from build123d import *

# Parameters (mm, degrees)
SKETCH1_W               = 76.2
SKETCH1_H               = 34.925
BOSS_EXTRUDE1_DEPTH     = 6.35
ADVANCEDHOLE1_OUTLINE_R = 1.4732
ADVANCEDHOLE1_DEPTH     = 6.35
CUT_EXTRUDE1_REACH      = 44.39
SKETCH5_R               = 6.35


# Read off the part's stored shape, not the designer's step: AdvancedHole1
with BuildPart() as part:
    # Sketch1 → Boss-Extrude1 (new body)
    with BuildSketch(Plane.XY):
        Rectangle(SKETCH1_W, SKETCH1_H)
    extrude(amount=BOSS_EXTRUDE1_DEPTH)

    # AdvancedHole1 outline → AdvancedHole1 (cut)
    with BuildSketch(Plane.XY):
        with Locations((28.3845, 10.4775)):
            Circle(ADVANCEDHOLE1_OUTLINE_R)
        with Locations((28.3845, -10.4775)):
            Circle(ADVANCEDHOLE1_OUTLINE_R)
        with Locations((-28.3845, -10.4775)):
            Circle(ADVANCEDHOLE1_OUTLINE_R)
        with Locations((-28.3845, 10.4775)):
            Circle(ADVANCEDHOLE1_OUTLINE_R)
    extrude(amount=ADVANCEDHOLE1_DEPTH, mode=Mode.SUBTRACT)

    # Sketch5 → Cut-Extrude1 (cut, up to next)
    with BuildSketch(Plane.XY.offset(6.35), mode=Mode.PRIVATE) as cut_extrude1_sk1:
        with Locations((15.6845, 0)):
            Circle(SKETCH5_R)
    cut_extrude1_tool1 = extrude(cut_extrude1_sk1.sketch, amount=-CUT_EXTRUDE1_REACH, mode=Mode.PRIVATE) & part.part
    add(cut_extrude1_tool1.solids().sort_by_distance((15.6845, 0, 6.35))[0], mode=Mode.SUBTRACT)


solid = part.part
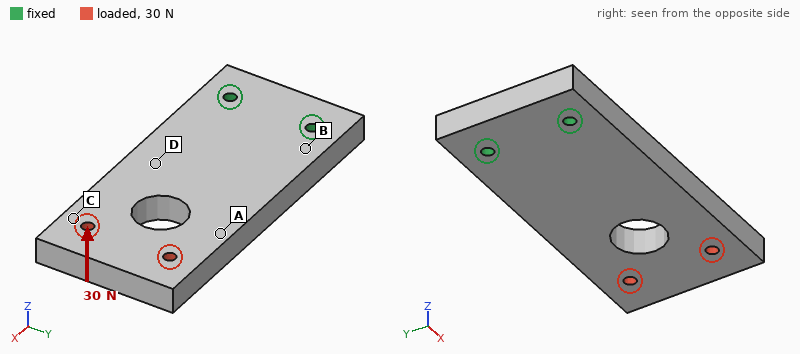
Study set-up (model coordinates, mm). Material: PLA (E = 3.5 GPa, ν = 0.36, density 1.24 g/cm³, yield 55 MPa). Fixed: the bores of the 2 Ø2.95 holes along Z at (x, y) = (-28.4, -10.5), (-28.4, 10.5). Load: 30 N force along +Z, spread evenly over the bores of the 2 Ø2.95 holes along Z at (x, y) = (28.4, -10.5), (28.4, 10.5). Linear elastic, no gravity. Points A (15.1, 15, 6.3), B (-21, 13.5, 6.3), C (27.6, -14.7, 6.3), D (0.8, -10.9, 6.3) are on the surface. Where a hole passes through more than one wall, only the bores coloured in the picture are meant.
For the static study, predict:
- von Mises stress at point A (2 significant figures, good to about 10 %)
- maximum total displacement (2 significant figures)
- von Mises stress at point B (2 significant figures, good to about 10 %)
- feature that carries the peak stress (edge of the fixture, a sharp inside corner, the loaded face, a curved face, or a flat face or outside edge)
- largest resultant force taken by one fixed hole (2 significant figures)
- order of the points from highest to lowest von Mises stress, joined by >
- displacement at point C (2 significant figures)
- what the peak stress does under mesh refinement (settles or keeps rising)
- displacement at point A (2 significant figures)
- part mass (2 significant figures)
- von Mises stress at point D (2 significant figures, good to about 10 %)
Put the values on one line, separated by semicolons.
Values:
2.4 MPa; 0.97 mm; 6.4 MPa; edge of the fixture; 15 N; B > D > A > C; 0.75 mm; keeps rising; 0.50 mm; 20 g; 3.7 MPa
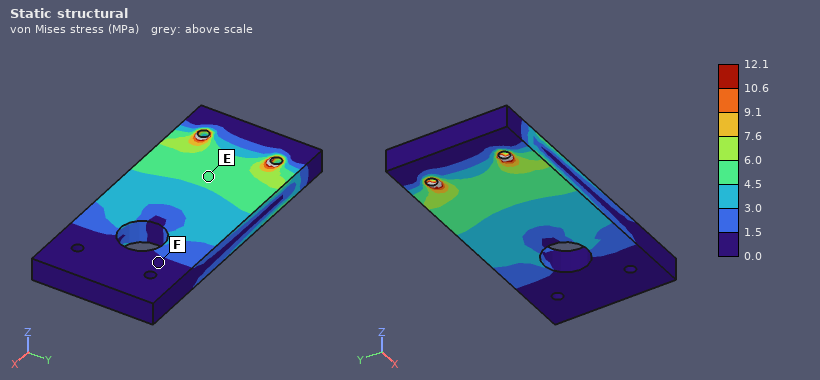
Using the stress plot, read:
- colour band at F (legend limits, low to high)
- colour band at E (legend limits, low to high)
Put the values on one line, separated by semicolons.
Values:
0.0 to 1.5 MPa; 4.5 to 6.0 MPa
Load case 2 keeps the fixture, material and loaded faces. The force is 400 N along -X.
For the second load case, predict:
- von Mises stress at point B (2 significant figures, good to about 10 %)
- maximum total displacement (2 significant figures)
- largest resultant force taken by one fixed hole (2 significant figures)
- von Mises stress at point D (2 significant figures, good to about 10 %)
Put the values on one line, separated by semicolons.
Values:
2.1 MPa; 42 µm; 200 N; 2.1 MPa
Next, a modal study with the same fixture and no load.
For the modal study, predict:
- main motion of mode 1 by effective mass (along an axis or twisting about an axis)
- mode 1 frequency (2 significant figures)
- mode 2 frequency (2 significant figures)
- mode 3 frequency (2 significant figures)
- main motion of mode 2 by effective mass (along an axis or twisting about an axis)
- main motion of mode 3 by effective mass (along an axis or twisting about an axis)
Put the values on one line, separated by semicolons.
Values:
along Z; 390 Hz; 1400 Hz; 1700 Hz; twisting about X; along Y
